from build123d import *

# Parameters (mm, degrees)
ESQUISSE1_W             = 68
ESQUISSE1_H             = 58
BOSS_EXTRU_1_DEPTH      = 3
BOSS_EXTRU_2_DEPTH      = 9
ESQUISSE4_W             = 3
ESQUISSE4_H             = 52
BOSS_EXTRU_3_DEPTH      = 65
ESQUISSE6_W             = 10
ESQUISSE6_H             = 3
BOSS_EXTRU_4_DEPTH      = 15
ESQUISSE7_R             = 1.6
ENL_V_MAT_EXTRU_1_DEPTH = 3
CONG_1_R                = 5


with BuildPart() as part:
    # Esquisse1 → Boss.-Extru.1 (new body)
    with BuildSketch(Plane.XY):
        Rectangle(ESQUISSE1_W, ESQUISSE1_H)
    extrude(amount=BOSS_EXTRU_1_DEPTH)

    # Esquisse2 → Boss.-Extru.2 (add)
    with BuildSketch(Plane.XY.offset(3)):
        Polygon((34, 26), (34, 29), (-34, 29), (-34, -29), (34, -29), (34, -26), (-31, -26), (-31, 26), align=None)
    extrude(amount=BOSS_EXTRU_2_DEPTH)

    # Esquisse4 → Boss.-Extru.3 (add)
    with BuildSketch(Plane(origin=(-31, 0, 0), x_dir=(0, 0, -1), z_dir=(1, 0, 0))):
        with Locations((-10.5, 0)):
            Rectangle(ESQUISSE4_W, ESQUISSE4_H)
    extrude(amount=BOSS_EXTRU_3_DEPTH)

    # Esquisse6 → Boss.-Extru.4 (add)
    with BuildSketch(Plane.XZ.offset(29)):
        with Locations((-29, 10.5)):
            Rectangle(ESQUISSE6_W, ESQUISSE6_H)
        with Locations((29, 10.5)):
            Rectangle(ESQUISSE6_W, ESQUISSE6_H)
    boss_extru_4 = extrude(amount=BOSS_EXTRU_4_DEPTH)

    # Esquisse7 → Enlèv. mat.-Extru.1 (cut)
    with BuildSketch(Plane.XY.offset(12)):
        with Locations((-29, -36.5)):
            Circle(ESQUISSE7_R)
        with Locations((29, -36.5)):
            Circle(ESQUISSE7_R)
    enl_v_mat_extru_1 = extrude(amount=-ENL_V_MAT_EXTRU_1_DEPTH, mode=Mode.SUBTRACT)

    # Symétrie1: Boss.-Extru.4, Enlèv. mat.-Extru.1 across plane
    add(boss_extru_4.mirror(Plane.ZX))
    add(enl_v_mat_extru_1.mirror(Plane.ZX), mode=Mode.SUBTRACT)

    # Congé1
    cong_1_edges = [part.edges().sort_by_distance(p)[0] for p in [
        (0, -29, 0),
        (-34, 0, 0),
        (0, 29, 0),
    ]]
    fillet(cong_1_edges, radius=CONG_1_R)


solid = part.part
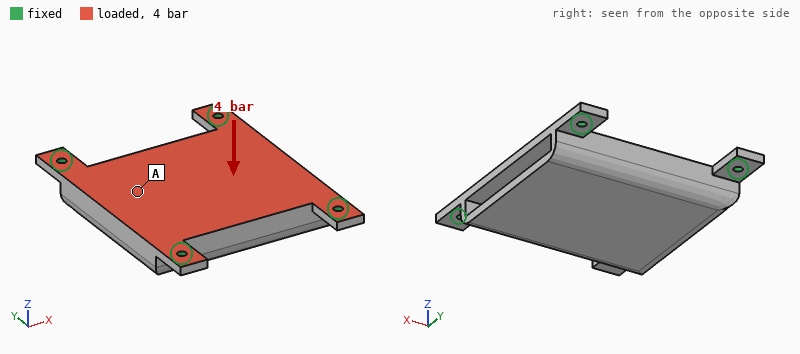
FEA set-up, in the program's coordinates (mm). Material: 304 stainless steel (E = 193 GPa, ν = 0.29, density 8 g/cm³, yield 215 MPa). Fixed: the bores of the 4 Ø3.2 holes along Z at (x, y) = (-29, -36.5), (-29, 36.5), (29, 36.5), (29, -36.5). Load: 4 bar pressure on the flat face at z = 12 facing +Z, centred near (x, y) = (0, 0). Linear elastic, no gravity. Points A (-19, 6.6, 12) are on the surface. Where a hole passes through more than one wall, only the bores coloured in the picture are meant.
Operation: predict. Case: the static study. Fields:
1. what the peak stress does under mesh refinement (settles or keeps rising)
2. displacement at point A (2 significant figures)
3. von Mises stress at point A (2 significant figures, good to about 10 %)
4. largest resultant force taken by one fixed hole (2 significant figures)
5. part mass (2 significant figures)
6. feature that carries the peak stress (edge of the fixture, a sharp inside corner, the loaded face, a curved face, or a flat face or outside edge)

keeps rising
21 µm
17 MPa
540 N
220 g
edge of the fixture
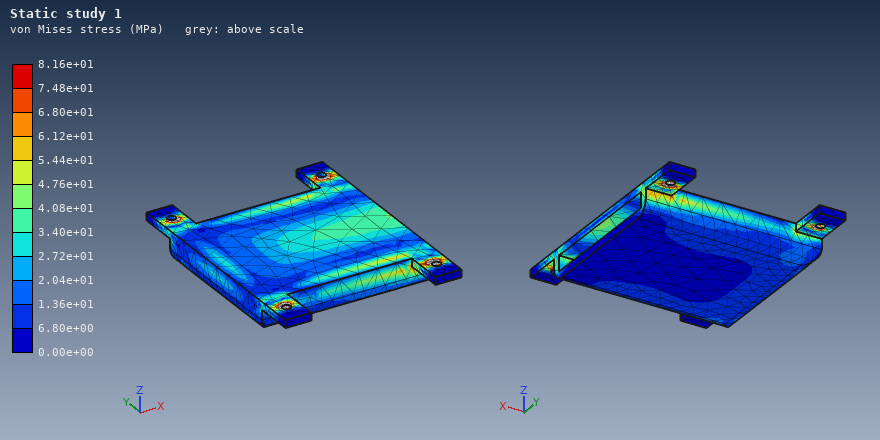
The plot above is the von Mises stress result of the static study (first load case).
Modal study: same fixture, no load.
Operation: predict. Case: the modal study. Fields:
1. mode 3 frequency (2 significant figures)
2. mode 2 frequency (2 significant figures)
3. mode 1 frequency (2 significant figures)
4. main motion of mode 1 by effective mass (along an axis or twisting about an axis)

4900 Hz
4400 Hz
3500 Hz
along Z
